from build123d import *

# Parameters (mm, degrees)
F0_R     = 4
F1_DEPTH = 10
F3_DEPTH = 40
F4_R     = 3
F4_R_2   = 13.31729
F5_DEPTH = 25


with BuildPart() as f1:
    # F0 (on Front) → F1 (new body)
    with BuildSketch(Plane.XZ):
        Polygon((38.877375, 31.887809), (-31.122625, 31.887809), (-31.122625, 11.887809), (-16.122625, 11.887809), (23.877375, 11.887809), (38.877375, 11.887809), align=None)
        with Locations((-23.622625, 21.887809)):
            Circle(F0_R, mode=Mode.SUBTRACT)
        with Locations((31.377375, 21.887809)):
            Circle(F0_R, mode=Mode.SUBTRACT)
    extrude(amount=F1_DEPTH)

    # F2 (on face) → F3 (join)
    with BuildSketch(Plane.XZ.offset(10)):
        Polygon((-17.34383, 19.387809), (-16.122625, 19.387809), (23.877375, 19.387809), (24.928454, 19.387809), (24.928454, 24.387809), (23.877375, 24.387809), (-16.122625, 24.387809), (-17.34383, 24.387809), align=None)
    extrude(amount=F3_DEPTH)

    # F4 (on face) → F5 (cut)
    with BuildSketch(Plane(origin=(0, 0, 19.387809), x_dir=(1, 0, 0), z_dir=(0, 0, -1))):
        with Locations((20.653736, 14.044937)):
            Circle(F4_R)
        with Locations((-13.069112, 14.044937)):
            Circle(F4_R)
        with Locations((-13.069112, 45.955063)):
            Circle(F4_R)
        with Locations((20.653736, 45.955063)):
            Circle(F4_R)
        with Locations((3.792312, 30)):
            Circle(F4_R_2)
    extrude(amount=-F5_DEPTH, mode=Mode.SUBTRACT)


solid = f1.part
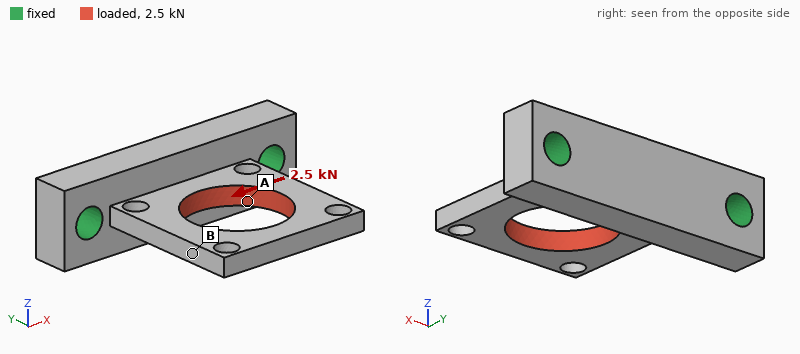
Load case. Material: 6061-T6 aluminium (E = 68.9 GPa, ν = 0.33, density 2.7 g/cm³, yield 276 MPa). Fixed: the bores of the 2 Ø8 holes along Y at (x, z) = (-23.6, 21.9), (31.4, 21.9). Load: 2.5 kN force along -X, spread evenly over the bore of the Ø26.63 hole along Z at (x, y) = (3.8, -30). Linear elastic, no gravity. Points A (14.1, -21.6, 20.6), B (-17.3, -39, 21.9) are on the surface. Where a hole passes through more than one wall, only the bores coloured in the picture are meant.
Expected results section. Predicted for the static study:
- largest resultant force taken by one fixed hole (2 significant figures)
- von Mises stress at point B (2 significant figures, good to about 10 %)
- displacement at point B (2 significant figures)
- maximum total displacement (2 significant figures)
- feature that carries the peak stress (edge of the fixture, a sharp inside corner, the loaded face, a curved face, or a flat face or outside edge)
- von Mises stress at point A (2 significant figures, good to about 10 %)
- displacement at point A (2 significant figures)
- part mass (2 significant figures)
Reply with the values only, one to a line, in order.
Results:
1.9 kN
31 MPa
0.096 mm
0.11 mm
a curved face
100 MPa
0.022 mm
49 g
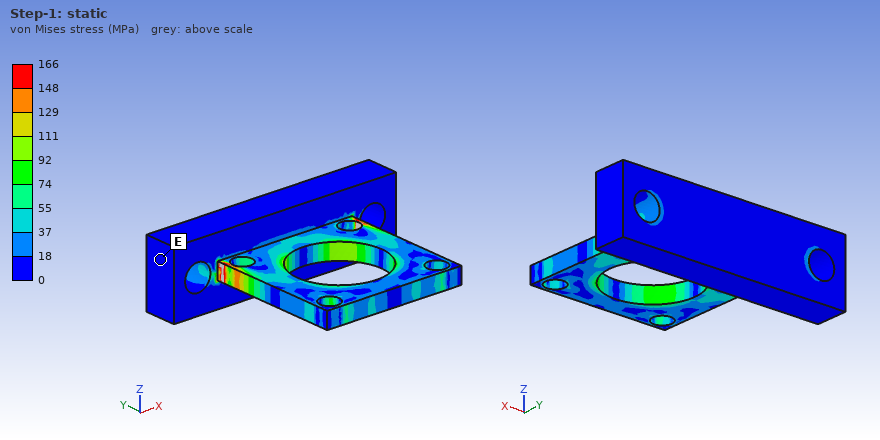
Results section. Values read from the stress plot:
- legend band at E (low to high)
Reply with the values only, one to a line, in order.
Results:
0 to 18 MPa
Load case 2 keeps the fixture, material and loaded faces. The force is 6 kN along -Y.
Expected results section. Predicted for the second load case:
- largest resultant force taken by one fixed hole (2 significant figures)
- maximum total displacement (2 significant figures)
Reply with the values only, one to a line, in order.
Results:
3.1 kN
66 µm
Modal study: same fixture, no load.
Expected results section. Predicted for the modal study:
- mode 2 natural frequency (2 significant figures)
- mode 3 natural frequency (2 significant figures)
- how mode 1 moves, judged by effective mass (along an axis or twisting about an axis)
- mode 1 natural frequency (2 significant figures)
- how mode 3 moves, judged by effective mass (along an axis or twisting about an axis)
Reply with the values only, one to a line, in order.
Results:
4300 Hz
7000 Hz
along Z
1900 Hz
along X
